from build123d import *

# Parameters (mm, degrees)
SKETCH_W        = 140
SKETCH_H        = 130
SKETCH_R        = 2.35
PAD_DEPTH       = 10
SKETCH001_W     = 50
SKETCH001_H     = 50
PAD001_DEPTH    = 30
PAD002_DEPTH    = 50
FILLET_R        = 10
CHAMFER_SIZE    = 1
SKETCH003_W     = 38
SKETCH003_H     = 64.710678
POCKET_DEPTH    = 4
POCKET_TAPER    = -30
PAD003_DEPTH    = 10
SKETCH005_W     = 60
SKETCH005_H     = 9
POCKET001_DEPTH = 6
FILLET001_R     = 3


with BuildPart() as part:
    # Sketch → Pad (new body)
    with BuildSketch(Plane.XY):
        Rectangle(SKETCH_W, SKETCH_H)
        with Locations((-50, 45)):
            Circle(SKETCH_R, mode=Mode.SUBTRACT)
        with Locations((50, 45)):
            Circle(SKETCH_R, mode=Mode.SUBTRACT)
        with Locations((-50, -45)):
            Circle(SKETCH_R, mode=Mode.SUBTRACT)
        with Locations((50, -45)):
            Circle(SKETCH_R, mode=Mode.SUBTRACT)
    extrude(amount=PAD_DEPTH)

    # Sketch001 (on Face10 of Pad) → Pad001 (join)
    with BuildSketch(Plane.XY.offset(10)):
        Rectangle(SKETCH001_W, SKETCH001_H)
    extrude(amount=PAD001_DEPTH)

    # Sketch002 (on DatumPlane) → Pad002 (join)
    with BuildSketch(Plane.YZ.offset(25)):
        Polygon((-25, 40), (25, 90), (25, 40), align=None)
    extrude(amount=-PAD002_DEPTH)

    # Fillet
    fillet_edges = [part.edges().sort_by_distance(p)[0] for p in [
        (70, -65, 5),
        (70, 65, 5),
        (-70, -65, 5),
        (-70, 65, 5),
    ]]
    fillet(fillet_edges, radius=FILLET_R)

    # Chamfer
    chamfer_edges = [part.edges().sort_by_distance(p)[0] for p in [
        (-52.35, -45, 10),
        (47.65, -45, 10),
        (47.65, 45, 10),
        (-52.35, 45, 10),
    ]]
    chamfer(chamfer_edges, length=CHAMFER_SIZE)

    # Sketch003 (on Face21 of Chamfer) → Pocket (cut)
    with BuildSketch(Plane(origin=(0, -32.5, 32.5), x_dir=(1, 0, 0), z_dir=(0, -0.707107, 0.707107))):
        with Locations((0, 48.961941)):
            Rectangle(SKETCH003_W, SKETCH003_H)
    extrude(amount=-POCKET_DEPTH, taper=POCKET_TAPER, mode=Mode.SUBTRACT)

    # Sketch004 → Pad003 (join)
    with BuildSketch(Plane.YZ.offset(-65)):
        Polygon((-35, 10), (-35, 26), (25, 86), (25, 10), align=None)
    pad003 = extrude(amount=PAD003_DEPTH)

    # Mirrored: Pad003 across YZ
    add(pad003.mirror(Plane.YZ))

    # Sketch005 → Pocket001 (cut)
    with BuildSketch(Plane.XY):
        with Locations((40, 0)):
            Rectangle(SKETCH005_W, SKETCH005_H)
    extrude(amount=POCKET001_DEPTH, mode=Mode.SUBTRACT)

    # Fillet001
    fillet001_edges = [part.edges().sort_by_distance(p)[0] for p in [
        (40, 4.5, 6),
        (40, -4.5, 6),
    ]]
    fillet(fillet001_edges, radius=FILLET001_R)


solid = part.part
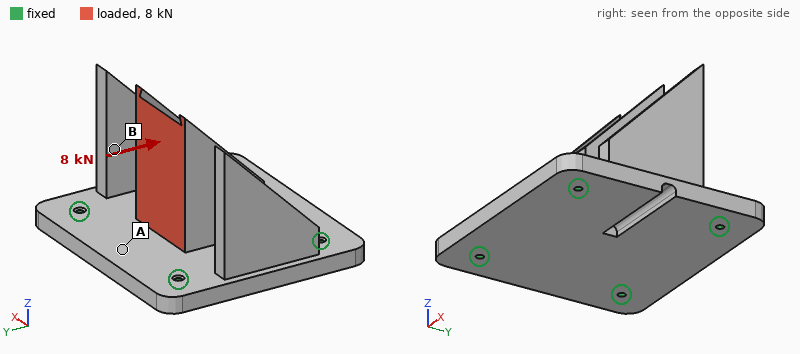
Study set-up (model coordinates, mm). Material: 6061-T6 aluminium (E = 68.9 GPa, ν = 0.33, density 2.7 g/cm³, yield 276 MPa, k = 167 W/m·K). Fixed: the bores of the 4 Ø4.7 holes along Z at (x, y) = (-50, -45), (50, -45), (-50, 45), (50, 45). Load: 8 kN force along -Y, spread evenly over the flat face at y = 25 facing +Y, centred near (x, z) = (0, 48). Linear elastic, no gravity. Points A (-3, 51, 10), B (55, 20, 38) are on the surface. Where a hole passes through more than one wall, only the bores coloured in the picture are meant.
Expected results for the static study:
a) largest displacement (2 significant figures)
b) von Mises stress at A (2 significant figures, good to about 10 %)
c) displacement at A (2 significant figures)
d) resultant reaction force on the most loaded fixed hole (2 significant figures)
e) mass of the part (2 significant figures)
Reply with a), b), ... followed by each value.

a) 0.21 mm
b) 21 MPa
c) 0.057 mm
d) 3.1 kN
e) 970 g
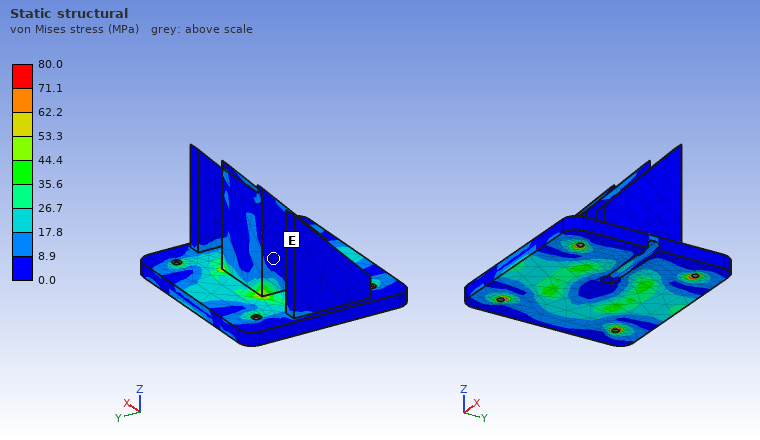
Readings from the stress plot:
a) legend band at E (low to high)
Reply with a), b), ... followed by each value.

a) 0.0 to 8.9 MPa
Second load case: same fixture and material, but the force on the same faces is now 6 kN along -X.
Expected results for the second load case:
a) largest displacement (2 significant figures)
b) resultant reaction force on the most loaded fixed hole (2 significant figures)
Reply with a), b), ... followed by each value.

a) 0.14 mm
b) 2.6 kN
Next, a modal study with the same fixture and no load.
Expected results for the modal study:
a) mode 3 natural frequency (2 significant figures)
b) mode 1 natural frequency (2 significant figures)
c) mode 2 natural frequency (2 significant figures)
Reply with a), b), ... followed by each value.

a) 2500 Hz
b) 1700 Hz
c) 1800 Hz
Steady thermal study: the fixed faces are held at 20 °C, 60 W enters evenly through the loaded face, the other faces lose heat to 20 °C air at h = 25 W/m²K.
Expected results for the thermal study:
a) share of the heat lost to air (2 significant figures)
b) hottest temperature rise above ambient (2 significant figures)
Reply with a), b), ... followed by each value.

a) 14 %
b) 18 K
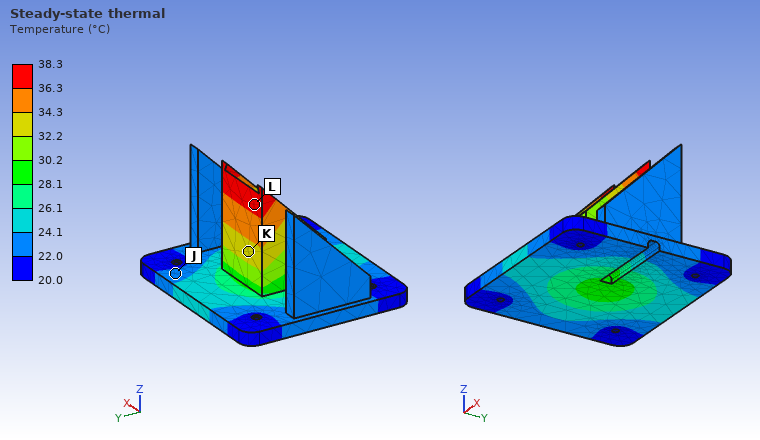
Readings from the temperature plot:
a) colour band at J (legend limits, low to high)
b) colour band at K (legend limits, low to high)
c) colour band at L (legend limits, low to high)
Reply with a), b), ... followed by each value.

a) 22.0 to 24.1 °C
b) 32.2 to 34.3 °C
c) 36.3 to 38.3 °C
